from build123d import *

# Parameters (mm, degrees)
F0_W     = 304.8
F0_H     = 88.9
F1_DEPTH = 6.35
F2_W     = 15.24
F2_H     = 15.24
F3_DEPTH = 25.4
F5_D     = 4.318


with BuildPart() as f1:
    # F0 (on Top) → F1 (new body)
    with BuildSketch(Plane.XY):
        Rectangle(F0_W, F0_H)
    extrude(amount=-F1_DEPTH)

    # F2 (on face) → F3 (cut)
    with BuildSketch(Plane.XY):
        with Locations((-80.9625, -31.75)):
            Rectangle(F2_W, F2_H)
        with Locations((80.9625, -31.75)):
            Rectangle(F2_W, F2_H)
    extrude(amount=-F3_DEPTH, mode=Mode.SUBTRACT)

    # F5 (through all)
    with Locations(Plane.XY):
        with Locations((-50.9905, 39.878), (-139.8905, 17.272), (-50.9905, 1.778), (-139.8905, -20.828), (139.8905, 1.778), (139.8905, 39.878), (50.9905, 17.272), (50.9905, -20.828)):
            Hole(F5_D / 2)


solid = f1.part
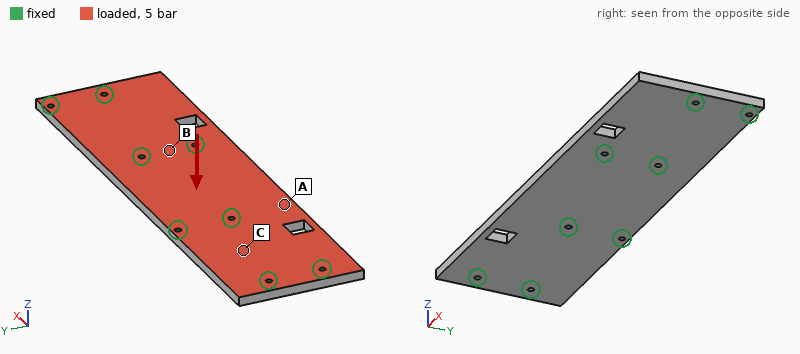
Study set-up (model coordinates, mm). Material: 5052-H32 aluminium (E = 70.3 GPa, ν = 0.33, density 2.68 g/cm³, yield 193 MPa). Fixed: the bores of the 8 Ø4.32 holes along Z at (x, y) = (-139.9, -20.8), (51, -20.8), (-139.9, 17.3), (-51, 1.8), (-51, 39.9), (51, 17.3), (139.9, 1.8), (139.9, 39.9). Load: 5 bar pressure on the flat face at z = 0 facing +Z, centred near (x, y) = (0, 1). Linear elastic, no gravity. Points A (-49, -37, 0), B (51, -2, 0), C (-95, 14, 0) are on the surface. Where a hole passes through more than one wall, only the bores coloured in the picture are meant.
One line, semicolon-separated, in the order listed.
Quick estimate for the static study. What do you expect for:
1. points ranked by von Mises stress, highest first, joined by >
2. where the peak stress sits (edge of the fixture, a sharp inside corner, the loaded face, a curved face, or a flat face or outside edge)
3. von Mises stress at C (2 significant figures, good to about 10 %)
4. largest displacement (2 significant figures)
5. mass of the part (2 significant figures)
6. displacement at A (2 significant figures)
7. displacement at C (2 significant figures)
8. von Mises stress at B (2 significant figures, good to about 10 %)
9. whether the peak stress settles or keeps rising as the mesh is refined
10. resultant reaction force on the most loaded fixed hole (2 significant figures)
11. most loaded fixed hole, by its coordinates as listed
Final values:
B > C > A; edge of the fixture; 26 MPa; 0.25 mm; 450 g; 0.19 mm; 0.059 mm; 40 MPa; keeps rising; 3.3 kN; (-51, 1.8)
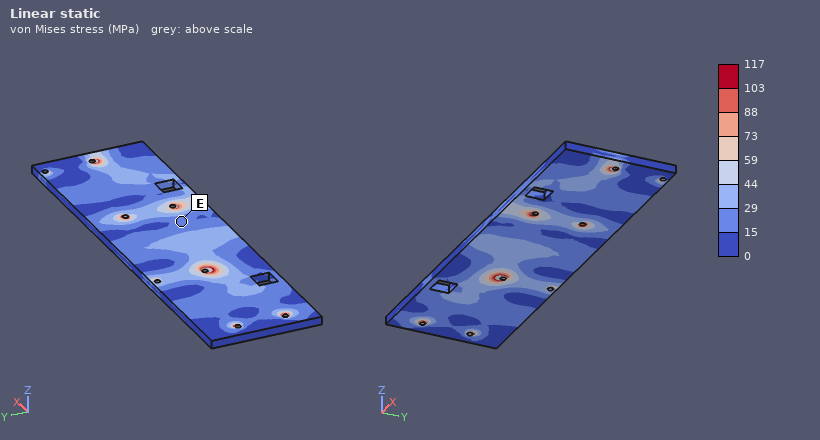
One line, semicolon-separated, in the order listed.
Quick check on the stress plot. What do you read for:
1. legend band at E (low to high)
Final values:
15 to 29 MPa
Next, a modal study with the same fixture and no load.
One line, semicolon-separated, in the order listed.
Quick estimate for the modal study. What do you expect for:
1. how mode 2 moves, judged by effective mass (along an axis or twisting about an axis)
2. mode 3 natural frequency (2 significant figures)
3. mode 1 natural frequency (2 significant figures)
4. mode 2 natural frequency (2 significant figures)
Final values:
along Z; 2800 Hz; 2200 Hz; 2400 Hz
